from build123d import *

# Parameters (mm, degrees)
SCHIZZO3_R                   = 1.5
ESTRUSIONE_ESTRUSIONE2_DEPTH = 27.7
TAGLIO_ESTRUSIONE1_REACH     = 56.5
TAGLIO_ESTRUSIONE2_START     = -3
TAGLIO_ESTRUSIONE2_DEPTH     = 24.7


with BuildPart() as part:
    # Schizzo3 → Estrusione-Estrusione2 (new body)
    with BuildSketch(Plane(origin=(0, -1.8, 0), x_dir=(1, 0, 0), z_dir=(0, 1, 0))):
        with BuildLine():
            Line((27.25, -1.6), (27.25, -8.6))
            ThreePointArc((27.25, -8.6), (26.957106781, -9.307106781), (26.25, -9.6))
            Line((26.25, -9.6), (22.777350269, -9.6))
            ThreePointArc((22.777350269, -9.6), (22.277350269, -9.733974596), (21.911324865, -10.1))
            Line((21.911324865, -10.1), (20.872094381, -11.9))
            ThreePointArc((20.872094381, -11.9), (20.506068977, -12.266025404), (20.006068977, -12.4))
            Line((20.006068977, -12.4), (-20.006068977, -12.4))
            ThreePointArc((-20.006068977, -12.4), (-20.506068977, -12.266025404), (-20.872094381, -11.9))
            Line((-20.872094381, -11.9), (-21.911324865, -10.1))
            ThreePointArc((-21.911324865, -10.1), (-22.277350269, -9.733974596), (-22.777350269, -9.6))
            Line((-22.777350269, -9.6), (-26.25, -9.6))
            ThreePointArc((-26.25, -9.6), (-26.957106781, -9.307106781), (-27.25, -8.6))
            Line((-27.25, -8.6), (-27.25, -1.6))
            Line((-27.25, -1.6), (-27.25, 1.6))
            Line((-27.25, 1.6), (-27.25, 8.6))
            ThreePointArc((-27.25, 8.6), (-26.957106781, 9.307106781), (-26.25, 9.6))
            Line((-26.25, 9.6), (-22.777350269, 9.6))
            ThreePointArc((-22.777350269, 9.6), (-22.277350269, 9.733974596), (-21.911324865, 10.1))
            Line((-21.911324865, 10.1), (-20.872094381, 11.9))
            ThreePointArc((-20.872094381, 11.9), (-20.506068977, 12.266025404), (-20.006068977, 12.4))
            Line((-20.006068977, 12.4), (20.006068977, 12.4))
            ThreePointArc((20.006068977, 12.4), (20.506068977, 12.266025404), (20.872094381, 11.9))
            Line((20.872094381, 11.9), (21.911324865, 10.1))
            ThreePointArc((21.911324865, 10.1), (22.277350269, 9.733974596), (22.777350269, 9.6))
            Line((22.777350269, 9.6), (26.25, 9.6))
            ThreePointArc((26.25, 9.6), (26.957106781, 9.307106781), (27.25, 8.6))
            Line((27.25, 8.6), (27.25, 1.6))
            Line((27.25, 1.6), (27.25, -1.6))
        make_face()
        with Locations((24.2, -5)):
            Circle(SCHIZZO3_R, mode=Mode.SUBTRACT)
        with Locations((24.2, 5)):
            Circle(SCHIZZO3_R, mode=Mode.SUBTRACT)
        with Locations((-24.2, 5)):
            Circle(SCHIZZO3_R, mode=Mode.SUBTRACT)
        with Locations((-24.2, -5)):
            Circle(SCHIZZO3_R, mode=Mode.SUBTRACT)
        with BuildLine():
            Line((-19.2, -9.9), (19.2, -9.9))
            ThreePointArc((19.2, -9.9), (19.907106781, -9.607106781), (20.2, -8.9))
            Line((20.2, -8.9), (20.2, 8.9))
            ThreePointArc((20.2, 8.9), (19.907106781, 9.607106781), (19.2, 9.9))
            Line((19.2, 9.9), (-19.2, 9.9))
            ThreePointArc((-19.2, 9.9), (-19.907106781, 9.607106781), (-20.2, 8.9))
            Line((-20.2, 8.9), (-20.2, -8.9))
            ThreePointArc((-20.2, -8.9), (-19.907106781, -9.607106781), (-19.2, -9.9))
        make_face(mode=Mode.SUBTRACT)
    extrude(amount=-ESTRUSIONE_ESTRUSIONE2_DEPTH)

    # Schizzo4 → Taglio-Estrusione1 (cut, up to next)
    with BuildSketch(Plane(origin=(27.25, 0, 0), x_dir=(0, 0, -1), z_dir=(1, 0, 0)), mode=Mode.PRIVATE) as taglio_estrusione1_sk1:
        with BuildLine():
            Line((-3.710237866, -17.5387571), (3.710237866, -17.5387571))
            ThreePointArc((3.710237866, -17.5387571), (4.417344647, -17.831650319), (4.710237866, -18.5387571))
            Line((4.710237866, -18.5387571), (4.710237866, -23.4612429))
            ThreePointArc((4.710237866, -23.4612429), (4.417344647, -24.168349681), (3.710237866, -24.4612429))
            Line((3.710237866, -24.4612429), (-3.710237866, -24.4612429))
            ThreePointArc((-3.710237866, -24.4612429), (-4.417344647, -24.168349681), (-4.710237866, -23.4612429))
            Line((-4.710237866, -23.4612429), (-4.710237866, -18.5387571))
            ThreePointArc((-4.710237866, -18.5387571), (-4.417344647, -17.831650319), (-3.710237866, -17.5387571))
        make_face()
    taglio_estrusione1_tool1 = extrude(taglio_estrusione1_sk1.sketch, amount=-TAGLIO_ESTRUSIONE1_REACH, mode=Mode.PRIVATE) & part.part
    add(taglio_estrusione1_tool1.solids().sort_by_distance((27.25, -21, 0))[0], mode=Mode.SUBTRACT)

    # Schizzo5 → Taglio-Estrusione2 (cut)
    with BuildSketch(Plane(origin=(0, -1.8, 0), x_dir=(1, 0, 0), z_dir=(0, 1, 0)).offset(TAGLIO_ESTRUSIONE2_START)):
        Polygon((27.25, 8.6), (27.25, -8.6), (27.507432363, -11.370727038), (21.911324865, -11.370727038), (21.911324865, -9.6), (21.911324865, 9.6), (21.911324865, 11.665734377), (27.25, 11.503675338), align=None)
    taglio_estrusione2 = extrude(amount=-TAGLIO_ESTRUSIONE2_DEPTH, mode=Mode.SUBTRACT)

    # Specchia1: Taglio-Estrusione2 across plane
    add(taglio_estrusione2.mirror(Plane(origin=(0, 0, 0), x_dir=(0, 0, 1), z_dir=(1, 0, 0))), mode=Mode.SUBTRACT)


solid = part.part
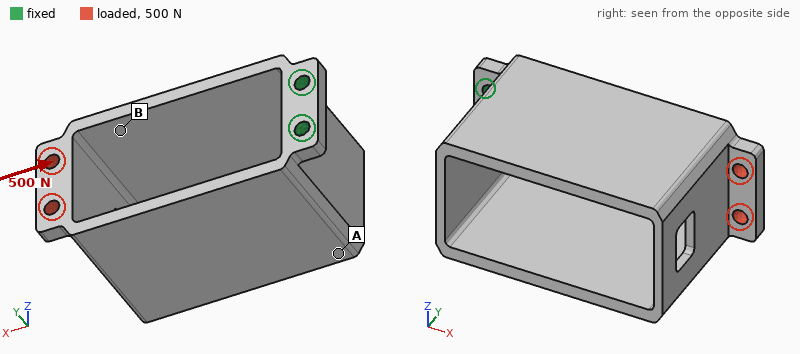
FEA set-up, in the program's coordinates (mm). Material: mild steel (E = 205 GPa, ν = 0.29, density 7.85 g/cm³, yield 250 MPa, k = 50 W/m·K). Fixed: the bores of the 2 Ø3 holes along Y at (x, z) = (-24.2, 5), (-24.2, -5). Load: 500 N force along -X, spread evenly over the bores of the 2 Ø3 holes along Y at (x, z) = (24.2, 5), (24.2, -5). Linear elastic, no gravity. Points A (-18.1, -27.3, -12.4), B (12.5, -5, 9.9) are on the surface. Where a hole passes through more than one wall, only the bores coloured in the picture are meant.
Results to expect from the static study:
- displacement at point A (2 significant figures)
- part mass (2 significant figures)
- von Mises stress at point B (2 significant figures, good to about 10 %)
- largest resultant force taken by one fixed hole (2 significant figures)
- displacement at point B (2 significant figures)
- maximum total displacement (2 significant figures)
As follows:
4.2 µm
64 g
26 MPa
280 N
16 µm
28 µm
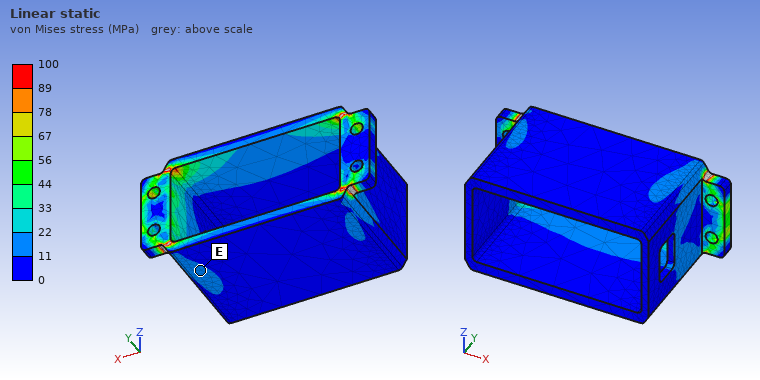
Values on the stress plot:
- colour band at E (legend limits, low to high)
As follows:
11 to 22 MPa
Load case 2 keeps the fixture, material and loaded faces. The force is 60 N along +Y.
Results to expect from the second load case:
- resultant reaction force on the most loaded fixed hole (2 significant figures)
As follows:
78 N
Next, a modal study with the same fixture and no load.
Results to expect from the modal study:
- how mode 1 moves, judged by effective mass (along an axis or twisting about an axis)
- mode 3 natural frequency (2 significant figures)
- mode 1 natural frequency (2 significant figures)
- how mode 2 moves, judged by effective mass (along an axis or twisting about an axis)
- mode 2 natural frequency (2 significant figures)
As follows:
along Y
2300 Hz
630 Hz
along Z
880 Hz
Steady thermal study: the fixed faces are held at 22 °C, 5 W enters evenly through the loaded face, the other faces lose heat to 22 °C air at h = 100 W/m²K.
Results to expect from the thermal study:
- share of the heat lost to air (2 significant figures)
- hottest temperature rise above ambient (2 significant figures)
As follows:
92 %
30 K
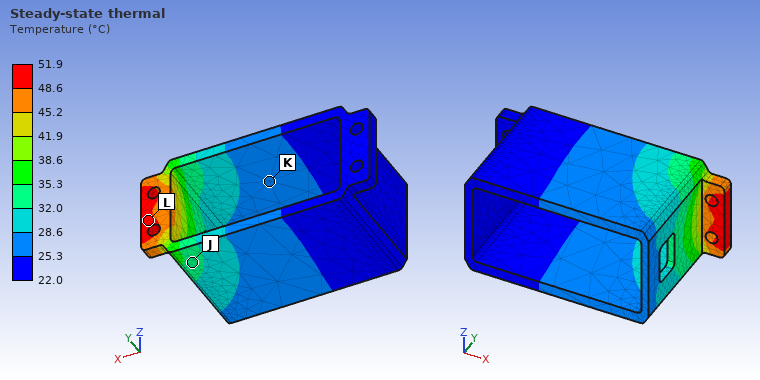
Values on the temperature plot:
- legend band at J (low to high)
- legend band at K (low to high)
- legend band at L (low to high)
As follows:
32.0 to 35.3 °C
25.3 to 28.6 °C
48.6 to 51.9 °C
